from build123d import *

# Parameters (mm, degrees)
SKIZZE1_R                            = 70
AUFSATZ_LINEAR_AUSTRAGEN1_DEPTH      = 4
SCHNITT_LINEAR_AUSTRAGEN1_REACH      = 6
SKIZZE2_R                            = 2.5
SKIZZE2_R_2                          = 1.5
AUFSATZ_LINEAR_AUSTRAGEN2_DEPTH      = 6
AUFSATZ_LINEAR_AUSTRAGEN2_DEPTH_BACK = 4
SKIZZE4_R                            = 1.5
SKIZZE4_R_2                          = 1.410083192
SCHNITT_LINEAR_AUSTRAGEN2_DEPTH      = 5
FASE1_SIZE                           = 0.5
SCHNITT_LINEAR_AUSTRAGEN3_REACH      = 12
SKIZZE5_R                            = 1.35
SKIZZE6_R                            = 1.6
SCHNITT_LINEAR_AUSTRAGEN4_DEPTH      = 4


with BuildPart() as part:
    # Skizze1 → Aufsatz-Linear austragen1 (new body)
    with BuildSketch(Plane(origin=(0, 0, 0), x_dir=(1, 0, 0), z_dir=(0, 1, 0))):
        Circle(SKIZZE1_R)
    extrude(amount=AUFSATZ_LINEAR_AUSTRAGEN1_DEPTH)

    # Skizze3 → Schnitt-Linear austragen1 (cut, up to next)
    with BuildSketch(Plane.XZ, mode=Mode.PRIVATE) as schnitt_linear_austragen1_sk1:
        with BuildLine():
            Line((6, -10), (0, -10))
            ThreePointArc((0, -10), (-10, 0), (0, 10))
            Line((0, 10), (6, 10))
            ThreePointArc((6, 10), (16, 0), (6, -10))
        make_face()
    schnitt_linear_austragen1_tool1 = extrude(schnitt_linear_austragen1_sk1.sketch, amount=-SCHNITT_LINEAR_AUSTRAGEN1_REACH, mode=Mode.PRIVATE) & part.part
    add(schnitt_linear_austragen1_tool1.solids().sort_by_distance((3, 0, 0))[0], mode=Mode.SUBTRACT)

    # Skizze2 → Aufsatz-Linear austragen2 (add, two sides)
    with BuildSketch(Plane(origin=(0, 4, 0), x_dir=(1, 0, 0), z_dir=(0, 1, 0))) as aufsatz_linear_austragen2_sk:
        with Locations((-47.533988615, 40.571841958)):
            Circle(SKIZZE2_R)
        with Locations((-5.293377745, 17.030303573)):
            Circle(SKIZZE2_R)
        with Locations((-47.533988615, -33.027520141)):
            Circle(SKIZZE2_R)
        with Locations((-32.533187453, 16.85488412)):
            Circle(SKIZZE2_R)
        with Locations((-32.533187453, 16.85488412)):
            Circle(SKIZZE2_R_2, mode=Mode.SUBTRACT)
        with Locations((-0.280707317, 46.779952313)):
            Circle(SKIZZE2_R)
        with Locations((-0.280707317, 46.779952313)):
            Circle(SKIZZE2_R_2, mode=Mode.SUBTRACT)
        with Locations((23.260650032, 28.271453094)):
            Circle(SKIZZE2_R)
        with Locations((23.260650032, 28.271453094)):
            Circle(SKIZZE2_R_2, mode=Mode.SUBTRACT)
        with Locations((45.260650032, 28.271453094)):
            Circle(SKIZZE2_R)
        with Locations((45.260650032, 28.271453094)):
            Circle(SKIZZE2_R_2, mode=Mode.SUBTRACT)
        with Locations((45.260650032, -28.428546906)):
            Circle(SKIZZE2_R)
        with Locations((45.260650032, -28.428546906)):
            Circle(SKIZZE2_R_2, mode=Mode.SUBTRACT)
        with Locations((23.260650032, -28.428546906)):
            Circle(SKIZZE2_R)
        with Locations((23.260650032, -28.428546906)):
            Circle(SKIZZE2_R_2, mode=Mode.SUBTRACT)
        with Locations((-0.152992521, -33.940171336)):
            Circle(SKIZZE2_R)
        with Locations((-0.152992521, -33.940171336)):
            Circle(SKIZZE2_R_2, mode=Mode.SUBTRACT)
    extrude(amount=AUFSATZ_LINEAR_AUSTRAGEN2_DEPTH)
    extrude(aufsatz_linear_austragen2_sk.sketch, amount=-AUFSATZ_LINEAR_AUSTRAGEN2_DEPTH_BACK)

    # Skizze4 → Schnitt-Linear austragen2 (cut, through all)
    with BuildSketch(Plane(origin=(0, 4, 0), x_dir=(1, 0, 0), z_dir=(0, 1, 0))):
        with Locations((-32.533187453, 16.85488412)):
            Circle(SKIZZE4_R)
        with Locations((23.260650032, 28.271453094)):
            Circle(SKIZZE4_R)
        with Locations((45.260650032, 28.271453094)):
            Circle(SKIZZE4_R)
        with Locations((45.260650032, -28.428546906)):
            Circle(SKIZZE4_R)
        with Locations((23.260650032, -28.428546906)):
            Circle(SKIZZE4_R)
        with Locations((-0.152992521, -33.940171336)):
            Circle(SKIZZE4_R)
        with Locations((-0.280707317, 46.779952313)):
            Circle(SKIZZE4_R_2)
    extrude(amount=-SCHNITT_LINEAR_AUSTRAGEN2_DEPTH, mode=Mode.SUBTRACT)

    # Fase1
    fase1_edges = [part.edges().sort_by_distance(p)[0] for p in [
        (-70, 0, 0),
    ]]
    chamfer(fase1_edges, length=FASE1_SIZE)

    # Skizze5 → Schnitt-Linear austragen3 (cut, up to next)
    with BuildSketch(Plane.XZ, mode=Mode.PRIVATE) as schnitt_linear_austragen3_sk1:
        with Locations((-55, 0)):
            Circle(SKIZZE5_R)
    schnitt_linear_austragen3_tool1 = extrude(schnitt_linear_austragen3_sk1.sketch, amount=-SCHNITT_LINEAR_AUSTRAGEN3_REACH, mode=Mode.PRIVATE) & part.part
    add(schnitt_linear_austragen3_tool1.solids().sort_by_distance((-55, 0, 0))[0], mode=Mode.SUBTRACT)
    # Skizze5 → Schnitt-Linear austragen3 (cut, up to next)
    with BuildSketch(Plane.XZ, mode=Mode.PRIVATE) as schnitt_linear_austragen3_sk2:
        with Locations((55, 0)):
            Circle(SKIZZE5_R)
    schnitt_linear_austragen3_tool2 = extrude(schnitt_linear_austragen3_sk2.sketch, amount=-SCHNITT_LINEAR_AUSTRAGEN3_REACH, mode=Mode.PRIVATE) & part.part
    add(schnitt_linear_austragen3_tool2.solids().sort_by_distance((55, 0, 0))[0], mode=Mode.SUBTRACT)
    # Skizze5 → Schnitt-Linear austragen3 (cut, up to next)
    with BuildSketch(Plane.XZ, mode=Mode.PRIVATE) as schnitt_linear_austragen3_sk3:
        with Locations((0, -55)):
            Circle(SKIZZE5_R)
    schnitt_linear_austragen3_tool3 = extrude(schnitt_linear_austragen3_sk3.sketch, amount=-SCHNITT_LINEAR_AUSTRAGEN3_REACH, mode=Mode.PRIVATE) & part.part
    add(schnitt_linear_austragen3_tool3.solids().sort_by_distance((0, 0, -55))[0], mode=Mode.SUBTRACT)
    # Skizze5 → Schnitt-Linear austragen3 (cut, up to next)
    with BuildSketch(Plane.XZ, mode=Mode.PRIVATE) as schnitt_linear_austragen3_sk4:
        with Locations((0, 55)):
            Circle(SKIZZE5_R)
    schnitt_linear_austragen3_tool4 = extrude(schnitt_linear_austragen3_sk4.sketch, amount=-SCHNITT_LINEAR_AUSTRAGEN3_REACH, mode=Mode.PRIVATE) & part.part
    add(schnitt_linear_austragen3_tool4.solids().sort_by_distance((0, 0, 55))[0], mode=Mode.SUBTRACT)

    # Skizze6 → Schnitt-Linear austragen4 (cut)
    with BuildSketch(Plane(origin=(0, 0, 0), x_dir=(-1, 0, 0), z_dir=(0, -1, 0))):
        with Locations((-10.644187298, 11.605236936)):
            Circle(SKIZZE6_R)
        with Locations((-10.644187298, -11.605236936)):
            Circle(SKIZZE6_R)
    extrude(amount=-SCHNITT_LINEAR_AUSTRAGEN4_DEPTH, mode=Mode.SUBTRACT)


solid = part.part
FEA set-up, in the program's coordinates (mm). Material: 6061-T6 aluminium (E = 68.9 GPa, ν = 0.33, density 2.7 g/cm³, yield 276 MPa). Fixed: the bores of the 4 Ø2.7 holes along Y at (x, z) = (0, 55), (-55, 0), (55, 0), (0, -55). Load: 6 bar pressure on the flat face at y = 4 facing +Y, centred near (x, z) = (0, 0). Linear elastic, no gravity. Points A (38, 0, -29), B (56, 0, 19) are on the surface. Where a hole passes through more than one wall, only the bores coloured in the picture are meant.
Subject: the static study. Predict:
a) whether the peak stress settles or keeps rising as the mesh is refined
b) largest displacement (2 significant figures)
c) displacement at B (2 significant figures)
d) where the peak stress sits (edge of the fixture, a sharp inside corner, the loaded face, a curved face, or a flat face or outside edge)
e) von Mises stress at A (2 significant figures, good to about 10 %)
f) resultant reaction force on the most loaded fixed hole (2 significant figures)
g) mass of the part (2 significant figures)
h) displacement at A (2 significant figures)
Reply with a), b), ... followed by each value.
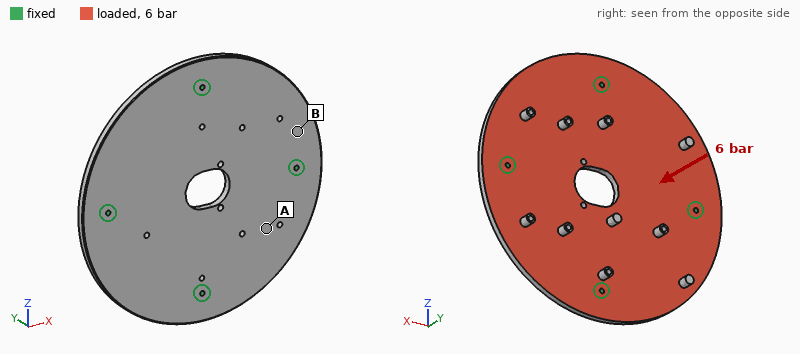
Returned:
a) keeps rising
b) 0.40 mm
c) 0.11 mm
d) edge of the fixture
e) 74 MPa
f) 2.2 kN
g) 160 g
h) 0.24 mm
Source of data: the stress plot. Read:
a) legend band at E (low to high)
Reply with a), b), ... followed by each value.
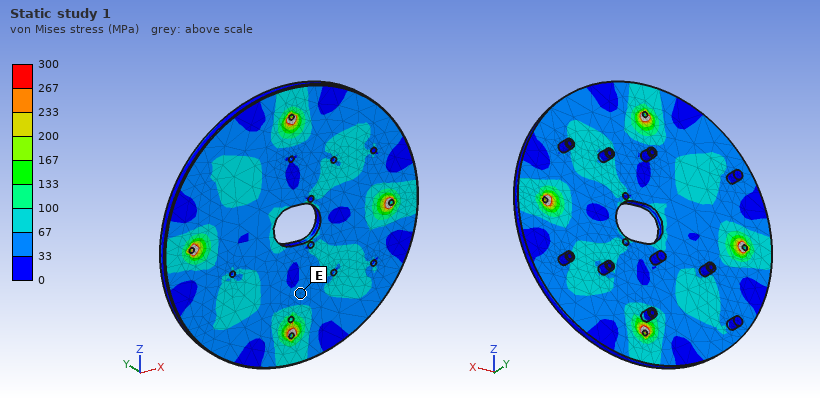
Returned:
a) 33 to 67 MPa
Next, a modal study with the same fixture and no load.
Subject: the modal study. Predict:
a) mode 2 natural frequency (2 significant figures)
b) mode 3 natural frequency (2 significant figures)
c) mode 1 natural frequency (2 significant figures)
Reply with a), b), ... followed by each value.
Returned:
a) 2200 Hz
b) 2200 Hz
c) 1900 Hz
